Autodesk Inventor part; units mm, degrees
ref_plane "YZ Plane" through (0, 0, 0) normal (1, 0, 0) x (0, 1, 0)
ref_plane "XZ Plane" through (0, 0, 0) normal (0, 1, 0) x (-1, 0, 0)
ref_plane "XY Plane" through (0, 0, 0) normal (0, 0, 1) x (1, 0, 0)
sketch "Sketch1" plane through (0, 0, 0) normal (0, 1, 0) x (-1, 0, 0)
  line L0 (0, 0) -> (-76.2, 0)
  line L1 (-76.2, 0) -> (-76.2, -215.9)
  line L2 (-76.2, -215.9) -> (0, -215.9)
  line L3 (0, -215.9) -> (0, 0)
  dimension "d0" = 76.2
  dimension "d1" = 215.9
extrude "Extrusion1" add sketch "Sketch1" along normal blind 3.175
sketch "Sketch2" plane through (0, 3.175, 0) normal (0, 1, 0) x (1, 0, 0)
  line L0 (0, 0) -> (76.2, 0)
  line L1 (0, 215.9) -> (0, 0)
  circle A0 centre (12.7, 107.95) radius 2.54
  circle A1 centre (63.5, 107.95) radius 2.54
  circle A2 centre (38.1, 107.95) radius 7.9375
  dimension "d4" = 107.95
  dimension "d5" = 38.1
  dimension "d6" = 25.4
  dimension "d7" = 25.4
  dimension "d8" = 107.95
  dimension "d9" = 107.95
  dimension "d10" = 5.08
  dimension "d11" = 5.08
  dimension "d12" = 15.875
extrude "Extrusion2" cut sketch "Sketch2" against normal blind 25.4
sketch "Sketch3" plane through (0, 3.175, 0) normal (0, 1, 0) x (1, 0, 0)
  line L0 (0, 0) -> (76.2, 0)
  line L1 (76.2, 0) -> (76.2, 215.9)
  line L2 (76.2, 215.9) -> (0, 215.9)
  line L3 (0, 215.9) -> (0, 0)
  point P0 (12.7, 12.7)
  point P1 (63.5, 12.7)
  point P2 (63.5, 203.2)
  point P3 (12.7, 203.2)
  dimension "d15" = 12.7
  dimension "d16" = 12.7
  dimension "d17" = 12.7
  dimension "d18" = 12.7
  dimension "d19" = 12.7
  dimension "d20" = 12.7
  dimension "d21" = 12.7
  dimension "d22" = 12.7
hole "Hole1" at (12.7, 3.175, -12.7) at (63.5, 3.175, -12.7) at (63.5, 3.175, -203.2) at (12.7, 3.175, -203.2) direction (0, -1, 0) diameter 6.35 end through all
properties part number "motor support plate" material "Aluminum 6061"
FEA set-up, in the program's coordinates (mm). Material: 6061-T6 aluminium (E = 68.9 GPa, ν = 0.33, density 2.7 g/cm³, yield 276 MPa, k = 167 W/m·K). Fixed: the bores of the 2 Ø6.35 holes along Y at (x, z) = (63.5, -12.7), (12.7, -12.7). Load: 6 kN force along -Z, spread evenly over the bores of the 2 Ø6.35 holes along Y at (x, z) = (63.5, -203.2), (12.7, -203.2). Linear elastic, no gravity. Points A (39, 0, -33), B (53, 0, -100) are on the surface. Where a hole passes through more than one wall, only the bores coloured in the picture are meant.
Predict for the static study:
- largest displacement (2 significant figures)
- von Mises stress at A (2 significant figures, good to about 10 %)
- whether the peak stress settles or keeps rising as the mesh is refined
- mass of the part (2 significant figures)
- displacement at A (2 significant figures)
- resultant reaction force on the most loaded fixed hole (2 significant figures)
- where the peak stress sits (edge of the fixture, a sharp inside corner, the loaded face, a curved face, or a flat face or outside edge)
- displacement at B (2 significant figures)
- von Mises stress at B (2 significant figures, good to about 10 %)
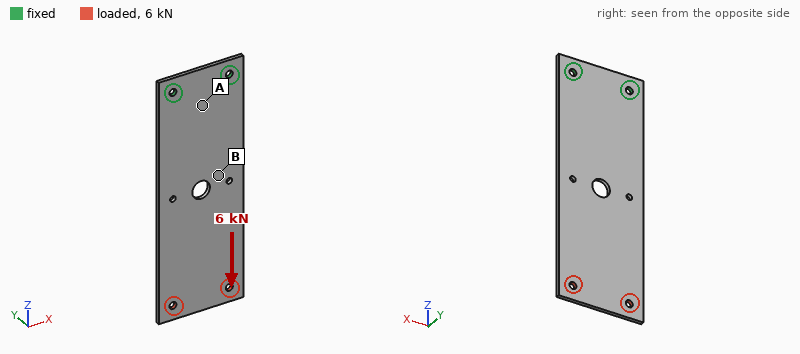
86 µm
15 MPa
keeps rising
140 g
13 µm
3.0 kN
edge of the fixture
37 µm
34 MPa
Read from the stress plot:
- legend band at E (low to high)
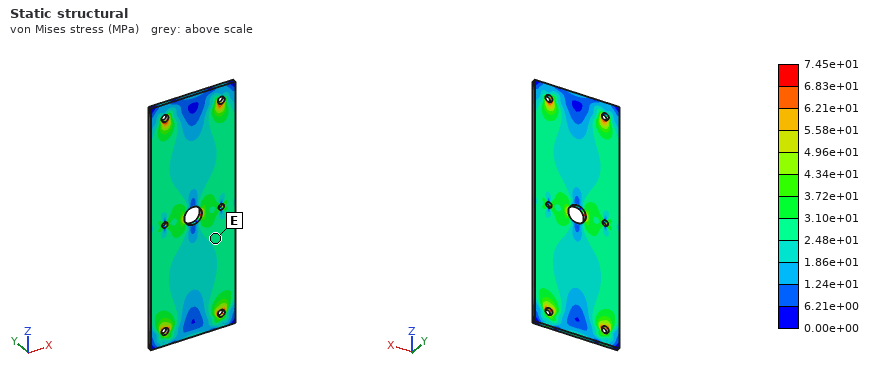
2.48e+01 to 3.10e+01 MPa
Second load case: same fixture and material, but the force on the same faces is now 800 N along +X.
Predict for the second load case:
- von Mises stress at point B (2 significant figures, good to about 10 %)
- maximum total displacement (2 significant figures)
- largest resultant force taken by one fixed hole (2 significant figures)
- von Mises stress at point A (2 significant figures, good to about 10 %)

15 MPa
0.32 mm
2.9 kN
9.2 MPa
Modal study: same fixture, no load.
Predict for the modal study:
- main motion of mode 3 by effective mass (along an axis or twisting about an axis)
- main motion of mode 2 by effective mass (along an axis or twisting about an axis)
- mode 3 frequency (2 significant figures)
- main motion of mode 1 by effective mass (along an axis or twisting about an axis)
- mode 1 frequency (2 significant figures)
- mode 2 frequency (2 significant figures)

along Y
twisting about Z
390 Hz
along Y
63 Hz
350 Hz
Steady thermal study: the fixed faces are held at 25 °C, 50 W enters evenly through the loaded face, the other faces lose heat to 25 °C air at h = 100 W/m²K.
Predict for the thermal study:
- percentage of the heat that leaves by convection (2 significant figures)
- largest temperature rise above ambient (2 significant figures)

97 %
59 K
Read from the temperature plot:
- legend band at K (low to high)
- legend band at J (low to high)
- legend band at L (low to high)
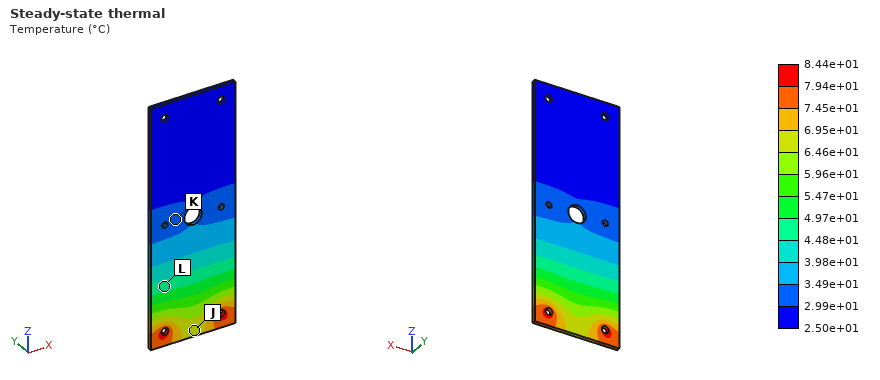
2.99e+01 to 3.49e+01 °C
6.46e+01 to 6.95e+01 °C
4.48e+01 to 4.97e+01 °C
